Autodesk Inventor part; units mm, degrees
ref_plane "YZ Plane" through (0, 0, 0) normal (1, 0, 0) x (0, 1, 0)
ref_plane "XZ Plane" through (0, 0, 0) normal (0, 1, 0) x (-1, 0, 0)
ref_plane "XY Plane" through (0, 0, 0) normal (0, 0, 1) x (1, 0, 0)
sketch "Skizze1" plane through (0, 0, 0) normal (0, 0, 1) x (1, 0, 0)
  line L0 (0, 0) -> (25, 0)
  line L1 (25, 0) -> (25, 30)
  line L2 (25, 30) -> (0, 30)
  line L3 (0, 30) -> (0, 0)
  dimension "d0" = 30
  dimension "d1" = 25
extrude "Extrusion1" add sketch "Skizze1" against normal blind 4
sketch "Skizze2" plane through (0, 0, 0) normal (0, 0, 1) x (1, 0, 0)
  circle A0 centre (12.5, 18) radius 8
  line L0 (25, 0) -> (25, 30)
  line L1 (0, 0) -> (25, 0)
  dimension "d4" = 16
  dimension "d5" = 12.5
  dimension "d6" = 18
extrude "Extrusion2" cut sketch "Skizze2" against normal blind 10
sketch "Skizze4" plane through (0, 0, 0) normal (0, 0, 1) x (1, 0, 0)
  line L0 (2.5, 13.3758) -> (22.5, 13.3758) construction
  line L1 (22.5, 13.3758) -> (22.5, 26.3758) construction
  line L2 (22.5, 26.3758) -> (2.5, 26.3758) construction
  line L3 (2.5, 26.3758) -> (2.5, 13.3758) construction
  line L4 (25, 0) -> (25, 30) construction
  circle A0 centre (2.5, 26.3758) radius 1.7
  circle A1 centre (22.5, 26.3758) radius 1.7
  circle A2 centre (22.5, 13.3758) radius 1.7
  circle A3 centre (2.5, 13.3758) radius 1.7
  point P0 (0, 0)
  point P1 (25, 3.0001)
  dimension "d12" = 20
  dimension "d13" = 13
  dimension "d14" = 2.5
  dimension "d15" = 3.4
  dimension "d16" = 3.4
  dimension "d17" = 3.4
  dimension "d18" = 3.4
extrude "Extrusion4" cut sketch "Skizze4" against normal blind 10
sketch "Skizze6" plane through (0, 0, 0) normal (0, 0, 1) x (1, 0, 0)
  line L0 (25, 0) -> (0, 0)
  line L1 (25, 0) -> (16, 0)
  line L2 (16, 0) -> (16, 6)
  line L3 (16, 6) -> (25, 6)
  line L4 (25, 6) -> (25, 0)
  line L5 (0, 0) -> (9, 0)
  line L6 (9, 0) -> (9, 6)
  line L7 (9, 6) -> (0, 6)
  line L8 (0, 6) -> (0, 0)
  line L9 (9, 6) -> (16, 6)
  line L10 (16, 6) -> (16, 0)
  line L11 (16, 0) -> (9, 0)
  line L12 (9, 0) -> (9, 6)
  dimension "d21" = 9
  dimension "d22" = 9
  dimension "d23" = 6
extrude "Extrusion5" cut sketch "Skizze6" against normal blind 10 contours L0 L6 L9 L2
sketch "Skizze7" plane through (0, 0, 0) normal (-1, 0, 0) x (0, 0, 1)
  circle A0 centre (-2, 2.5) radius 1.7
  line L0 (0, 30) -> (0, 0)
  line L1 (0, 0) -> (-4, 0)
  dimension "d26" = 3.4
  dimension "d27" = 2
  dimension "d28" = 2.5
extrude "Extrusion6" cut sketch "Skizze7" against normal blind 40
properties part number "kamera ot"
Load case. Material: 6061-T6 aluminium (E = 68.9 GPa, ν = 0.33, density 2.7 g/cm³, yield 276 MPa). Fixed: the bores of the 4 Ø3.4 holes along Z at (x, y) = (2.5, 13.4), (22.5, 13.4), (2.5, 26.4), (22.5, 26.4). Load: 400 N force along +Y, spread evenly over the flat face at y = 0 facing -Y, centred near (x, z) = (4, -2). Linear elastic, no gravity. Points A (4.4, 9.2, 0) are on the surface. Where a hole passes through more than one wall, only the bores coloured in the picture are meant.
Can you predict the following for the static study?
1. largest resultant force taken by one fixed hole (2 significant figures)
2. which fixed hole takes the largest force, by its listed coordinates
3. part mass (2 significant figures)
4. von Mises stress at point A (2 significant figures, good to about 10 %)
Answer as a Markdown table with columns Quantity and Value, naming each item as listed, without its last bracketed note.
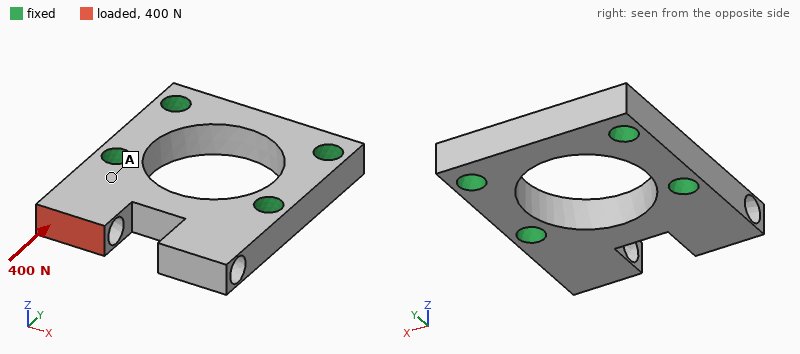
| Quantity | Value |
|---|---|
| largest resultant force taken by one fixed hole | 370 N |
| which fixed hole takes the largest force, by its listed coordinates | (2.5, 13.4) |
| part mass | 4.6 g |
| von Mises stress at point A | 15 MPa |
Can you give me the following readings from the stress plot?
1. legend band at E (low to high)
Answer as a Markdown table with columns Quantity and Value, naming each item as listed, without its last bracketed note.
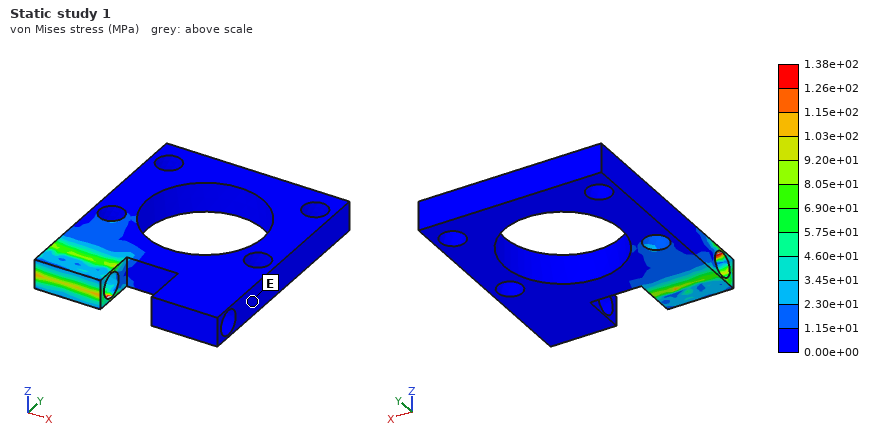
| Quantity | Value |
|---|---|
| legend band at E | 0.00e+00 to 1.15e+01 MPa |
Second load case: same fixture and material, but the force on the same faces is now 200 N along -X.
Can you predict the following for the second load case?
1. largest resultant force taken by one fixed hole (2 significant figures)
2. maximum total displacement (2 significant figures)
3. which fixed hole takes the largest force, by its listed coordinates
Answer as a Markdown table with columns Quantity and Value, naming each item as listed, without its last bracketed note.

| Quantity | Value |
|---|---|
| largest resultant force taken by one fixed hole | 200 N |
| maximum total displacement | 18 µm |
| which fixed hole takes the largest force, by its listed coordinates | (22.5, 13.4) |
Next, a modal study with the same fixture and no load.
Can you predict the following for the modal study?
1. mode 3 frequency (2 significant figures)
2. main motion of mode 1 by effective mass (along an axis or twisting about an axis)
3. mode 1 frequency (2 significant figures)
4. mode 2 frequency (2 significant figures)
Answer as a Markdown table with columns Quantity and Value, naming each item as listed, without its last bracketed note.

| Quantity | Value |
|---|---|
| mode 3 frequency | 40 kHz |
| main motion of mode 1 by effective mass | along Z |
| mode 1 frequency | 20 kHz |
| mode 2 frequency | 23 kHz |
